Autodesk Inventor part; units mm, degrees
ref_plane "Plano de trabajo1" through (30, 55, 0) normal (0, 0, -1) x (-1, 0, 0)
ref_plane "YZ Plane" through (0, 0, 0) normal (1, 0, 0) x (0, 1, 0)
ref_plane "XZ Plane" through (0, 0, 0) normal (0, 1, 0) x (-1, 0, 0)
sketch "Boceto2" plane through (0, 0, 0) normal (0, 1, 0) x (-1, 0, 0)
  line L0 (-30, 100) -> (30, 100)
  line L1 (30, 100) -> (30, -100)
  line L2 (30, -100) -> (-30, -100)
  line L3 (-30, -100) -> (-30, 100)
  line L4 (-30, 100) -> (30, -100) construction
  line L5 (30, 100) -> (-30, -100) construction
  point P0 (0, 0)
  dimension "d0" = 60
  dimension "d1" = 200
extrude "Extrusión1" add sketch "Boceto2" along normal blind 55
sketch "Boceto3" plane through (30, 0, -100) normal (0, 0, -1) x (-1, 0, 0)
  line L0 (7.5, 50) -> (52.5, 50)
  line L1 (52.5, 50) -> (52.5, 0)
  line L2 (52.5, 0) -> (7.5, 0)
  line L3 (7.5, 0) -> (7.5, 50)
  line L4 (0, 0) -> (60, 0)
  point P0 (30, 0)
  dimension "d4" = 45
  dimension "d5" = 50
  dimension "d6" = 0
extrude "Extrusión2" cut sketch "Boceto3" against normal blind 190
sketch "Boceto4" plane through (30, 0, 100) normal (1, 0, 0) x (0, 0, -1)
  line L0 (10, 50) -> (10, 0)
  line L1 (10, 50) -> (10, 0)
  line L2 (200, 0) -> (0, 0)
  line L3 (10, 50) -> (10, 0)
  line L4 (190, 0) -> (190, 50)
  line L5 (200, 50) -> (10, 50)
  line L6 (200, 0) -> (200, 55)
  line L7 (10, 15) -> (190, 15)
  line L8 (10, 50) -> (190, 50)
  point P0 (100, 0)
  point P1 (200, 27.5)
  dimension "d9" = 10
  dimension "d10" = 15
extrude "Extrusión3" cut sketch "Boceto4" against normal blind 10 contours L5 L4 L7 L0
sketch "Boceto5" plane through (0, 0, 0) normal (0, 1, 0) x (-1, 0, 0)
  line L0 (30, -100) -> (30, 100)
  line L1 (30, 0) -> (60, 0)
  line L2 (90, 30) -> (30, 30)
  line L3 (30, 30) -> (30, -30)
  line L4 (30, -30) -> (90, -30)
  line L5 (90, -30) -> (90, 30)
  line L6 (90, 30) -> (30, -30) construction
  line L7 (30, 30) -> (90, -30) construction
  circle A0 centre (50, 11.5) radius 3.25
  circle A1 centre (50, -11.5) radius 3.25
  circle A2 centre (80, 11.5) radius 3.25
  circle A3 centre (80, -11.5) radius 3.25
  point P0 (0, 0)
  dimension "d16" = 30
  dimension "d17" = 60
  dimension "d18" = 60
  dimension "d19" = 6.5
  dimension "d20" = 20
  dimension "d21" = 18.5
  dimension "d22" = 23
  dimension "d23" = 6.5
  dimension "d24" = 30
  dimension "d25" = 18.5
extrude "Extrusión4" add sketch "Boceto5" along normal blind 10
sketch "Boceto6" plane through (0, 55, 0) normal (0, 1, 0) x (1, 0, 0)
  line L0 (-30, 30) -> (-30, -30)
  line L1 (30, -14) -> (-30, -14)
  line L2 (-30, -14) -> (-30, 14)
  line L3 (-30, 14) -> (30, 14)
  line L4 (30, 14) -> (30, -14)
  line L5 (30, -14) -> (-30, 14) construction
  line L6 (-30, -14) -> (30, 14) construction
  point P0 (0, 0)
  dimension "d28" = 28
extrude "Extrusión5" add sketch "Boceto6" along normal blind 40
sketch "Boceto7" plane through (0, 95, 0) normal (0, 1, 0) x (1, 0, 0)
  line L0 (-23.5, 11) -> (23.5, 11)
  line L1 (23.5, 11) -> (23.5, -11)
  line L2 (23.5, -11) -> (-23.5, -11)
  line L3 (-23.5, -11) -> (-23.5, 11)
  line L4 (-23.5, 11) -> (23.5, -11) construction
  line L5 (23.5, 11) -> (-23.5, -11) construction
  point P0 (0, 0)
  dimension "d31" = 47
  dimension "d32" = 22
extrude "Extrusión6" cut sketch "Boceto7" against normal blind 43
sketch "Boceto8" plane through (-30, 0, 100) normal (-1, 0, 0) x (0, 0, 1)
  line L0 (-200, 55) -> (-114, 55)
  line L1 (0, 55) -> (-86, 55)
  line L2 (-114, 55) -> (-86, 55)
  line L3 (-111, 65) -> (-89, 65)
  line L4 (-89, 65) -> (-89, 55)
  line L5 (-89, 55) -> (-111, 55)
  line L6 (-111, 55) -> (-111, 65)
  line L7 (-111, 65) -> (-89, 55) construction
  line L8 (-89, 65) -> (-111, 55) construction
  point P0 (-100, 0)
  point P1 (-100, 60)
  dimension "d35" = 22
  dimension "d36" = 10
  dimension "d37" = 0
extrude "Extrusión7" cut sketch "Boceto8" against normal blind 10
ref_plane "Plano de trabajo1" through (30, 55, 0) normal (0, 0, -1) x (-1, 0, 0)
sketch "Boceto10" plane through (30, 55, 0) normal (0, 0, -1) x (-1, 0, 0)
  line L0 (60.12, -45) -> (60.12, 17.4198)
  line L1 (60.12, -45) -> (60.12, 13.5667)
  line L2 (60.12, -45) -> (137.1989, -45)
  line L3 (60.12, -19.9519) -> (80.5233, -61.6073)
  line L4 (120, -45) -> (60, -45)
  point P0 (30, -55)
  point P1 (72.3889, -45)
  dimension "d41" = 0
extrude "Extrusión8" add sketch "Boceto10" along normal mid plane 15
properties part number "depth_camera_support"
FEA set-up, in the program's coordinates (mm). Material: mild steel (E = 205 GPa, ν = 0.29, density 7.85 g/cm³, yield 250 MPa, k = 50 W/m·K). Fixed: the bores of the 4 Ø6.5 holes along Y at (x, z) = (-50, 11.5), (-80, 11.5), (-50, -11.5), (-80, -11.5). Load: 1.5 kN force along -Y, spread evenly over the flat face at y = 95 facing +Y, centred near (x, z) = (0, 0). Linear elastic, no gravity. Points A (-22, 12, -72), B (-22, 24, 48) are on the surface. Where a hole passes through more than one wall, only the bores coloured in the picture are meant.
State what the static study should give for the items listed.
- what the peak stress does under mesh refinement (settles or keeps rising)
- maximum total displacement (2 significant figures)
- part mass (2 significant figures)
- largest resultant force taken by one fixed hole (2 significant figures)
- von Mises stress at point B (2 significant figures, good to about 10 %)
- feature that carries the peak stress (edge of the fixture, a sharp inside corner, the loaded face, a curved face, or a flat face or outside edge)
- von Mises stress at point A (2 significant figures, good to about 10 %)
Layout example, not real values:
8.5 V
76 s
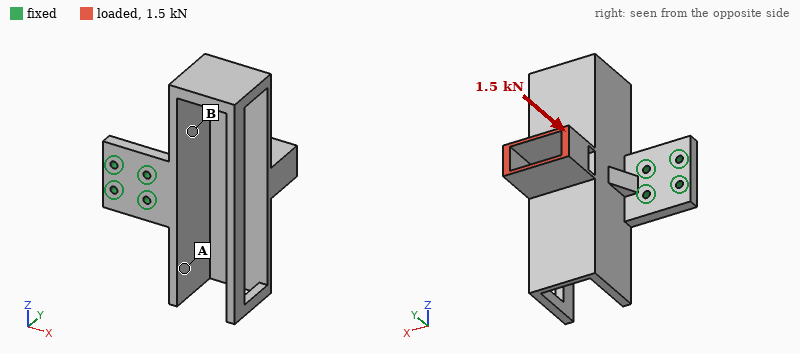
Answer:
keeps rising
0.37 mm
1.9 kg
1.1 kN
21 MPa
edge of the fixture
9.3 MPa
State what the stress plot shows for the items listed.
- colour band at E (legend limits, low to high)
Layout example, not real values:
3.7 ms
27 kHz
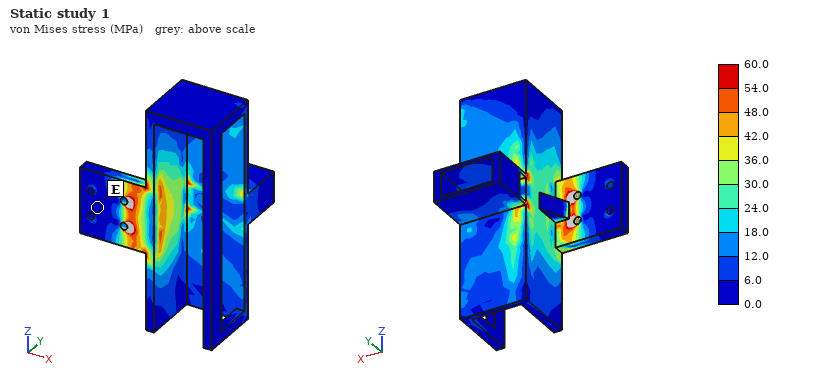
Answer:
0.0 to 6.0 MPa
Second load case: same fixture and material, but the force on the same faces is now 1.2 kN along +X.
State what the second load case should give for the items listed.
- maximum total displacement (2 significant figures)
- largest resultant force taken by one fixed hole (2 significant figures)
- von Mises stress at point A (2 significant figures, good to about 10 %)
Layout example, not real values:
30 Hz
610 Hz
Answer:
0.70 mm
820 N
18 MPa
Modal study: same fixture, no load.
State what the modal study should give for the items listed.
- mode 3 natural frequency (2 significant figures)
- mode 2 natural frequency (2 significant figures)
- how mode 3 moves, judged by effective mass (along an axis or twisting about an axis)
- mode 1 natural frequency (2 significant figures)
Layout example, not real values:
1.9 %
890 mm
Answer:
560 Hz
400 Hz
along X
330 Hz
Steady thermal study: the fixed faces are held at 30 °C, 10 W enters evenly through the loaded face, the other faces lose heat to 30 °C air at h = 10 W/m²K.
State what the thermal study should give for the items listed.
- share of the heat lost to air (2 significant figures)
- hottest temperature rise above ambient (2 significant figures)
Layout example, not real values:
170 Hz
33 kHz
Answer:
63 %
26 K
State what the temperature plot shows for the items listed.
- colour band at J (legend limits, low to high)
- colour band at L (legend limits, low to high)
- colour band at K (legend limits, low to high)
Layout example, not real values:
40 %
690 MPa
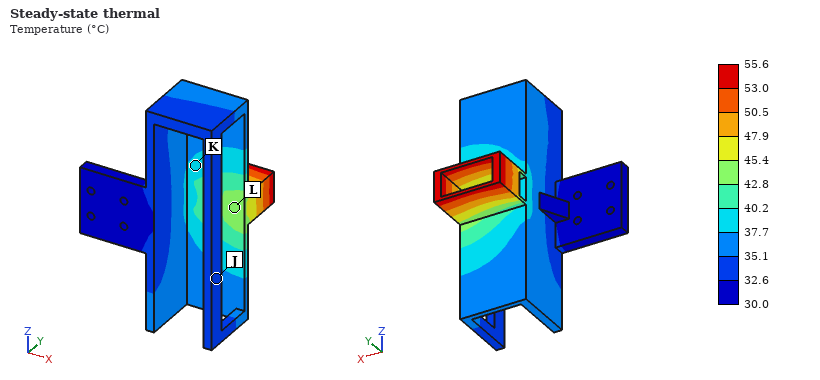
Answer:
32.6 to 35.1 °C
42.8 to 45.4 °C
37.7 to 40.2 °C
